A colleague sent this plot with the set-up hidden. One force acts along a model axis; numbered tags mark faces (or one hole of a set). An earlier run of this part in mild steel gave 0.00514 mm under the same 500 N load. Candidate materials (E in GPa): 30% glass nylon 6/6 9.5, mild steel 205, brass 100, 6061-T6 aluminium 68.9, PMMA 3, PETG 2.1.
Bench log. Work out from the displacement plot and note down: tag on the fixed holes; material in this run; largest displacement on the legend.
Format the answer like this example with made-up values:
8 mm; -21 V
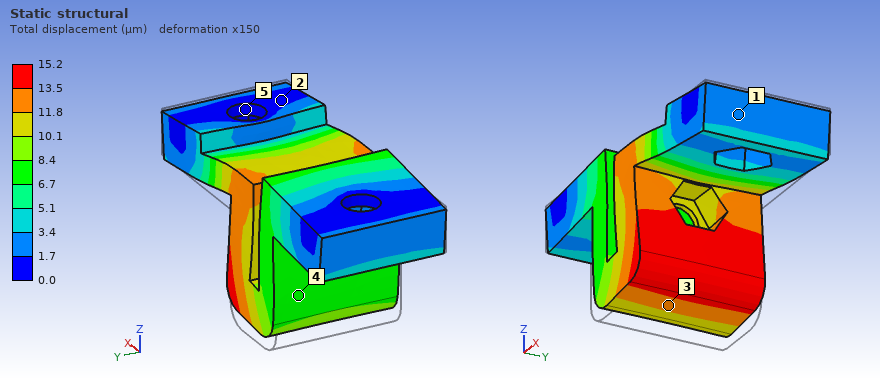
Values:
5; 6061-T6 aluminium; 15.2 µm
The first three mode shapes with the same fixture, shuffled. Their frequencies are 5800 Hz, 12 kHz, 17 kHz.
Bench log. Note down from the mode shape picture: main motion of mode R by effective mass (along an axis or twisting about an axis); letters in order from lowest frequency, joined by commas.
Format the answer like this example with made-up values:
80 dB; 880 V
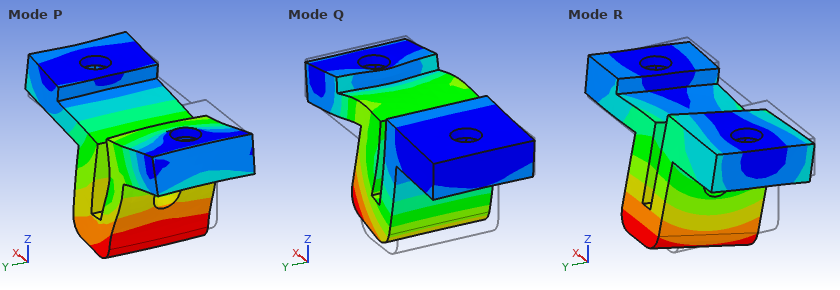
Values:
along Y; R, Q, P
